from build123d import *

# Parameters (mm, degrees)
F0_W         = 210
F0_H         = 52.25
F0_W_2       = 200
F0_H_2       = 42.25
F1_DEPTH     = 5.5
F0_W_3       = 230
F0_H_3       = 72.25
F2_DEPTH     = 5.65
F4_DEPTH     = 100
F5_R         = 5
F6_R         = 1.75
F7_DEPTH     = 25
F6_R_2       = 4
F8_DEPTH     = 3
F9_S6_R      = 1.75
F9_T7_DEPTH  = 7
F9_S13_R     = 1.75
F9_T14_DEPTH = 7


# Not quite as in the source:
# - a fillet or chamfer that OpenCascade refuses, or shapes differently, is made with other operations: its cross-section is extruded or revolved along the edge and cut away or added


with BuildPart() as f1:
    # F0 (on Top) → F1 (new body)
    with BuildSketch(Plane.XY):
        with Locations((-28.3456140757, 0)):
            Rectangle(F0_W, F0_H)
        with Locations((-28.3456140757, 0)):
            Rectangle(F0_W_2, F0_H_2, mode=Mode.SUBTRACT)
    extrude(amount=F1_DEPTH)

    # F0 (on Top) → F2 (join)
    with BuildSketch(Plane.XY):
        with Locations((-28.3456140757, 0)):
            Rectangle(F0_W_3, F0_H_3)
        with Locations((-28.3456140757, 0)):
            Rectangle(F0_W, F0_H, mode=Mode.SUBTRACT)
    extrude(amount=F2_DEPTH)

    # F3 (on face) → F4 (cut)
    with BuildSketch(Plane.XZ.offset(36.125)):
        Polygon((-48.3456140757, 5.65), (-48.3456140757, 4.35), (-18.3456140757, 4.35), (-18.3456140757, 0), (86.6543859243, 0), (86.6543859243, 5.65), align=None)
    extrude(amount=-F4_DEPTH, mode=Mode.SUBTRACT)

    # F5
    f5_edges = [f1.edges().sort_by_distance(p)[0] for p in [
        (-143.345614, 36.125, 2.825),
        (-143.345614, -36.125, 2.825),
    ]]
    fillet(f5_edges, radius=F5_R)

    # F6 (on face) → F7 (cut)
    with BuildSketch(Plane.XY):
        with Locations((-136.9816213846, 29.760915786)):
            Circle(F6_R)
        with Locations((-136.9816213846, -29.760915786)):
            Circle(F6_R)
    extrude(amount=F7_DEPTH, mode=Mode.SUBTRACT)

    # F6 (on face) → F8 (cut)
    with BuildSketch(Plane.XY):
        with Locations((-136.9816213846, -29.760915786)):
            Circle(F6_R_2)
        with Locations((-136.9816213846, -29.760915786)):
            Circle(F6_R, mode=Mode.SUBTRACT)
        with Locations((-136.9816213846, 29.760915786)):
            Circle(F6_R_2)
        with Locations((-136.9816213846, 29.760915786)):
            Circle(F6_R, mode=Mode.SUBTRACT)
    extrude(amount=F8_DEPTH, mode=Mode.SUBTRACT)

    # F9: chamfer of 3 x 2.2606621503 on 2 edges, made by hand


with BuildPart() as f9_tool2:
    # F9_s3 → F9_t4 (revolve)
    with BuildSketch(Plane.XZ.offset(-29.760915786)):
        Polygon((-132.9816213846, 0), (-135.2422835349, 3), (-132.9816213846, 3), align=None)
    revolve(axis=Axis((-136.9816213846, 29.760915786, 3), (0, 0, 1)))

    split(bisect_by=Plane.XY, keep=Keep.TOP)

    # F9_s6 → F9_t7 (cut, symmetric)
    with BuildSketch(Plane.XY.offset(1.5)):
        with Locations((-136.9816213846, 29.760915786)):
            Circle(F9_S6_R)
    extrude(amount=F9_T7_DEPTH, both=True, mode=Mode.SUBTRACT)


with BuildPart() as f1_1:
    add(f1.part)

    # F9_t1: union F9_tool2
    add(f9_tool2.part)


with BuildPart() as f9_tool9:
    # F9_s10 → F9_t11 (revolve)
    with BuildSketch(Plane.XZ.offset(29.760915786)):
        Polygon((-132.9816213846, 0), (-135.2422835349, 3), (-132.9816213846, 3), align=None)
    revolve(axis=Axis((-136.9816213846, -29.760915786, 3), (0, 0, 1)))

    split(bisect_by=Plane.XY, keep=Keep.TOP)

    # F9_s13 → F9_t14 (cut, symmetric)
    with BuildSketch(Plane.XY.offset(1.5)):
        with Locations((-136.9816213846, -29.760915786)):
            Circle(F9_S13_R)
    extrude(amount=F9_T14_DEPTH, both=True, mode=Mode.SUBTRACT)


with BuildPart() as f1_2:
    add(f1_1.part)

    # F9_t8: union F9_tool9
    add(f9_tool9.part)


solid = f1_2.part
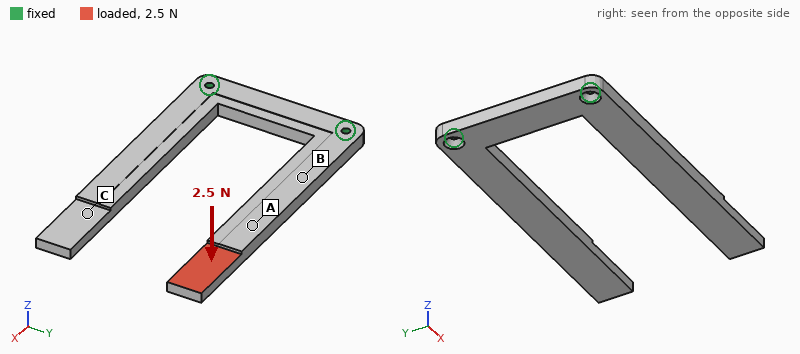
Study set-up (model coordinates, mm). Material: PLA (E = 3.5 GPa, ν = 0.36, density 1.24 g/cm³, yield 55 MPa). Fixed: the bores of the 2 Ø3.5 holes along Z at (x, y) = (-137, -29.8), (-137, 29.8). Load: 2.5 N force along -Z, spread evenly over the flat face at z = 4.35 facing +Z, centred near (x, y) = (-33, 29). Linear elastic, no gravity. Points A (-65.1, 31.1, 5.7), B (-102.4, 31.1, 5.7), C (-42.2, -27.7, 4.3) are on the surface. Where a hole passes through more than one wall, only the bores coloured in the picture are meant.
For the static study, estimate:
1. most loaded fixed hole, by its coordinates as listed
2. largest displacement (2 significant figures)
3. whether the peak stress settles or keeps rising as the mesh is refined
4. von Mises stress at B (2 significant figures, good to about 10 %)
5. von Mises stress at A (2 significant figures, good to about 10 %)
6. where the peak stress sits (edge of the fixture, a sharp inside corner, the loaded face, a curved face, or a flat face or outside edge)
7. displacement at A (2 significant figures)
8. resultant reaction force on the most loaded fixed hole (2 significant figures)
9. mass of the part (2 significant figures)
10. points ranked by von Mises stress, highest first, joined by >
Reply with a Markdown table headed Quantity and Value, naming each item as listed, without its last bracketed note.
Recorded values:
| Quantity | Value |
|---|---|
| most loaded fixed hole, by its coordinates as listed | (-137, 29.8) |
| largest displacement | 1.7 mm |
| whether the peak stress settles or keeps rising as the mesh is refined | keeps rising |
| von Mises stress at B | 2.2 MPa |
| von Mises stress at A | 1.0 MPa |
| where the peak stress sits | edge of the fixture |
| displacement at A | 0.79 mm |
| resultant reaction force on the most loaded fixed hole | 2.9 N |
| mass of the part | 29 g |
| points ranked by von Mises stress, highest first, joined by > | B > A > C |
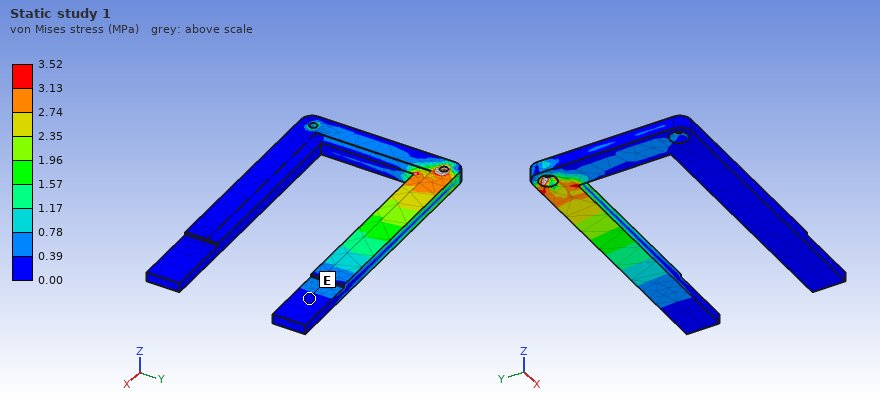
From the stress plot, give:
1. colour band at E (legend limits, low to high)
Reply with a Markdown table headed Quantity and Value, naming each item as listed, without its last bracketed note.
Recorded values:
| Quantity | Value |
|---|---|
| colour band at E | 0.00 to 0.39 MPa |
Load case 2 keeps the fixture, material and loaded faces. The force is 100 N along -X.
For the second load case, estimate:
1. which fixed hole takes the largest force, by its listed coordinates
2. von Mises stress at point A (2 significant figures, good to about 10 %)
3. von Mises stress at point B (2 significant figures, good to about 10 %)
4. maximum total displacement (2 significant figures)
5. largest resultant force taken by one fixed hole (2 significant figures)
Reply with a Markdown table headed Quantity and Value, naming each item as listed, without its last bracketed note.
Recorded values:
| Quantity | Value |
|---|---|
| which fixed hole takes the largest force, by its listed coordinates | (-137, 29.8) |
| von Mises stress at point A | 3.2 MPa |
| von Mises stress at point B | 3.2 MPa |
| maximum total displacement | 1.5 mm |
| largest resultant force taken by one fixed hole | 98 N |
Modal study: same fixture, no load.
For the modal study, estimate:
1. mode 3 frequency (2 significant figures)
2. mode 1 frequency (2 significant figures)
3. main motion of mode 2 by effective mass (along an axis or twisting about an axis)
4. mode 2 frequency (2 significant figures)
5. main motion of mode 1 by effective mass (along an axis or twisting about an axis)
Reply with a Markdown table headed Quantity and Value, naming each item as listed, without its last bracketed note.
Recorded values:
| Quantity | Value |
|---|---|
| mode 3 frequency | 260 Hz |
| mode 1 frequency | 110 Hz |
| main motion of mode 2 by effective mass | twisting about X |
| mode 2 frequency | 110 Hz |
| main motion of mode 1 by effective mass | along Z |
